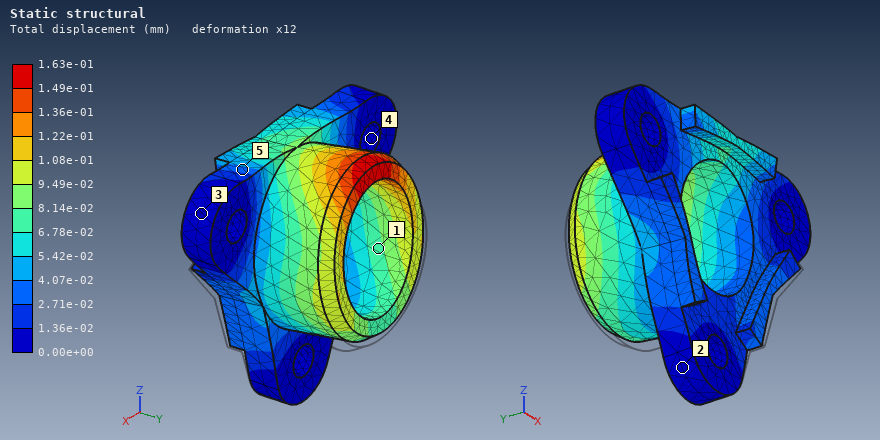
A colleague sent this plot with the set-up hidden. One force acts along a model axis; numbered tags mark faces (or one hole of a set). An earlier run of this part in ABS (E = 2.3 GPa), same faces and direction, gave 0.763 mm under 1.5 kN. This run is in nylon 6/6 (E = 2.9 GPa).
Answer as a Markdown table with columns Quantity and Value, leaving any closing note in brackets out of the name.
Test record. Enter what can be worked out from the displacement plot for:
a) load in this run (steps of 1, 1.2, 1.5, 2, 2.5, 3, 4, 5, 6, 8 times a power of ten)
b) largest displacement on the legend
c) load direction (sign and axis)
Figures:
| Quantity | Value |
|---|---|
| load in this run | 400 N |
| largest displacement on the legend | 1.63e-01 mm |
| load direction | +Z |
